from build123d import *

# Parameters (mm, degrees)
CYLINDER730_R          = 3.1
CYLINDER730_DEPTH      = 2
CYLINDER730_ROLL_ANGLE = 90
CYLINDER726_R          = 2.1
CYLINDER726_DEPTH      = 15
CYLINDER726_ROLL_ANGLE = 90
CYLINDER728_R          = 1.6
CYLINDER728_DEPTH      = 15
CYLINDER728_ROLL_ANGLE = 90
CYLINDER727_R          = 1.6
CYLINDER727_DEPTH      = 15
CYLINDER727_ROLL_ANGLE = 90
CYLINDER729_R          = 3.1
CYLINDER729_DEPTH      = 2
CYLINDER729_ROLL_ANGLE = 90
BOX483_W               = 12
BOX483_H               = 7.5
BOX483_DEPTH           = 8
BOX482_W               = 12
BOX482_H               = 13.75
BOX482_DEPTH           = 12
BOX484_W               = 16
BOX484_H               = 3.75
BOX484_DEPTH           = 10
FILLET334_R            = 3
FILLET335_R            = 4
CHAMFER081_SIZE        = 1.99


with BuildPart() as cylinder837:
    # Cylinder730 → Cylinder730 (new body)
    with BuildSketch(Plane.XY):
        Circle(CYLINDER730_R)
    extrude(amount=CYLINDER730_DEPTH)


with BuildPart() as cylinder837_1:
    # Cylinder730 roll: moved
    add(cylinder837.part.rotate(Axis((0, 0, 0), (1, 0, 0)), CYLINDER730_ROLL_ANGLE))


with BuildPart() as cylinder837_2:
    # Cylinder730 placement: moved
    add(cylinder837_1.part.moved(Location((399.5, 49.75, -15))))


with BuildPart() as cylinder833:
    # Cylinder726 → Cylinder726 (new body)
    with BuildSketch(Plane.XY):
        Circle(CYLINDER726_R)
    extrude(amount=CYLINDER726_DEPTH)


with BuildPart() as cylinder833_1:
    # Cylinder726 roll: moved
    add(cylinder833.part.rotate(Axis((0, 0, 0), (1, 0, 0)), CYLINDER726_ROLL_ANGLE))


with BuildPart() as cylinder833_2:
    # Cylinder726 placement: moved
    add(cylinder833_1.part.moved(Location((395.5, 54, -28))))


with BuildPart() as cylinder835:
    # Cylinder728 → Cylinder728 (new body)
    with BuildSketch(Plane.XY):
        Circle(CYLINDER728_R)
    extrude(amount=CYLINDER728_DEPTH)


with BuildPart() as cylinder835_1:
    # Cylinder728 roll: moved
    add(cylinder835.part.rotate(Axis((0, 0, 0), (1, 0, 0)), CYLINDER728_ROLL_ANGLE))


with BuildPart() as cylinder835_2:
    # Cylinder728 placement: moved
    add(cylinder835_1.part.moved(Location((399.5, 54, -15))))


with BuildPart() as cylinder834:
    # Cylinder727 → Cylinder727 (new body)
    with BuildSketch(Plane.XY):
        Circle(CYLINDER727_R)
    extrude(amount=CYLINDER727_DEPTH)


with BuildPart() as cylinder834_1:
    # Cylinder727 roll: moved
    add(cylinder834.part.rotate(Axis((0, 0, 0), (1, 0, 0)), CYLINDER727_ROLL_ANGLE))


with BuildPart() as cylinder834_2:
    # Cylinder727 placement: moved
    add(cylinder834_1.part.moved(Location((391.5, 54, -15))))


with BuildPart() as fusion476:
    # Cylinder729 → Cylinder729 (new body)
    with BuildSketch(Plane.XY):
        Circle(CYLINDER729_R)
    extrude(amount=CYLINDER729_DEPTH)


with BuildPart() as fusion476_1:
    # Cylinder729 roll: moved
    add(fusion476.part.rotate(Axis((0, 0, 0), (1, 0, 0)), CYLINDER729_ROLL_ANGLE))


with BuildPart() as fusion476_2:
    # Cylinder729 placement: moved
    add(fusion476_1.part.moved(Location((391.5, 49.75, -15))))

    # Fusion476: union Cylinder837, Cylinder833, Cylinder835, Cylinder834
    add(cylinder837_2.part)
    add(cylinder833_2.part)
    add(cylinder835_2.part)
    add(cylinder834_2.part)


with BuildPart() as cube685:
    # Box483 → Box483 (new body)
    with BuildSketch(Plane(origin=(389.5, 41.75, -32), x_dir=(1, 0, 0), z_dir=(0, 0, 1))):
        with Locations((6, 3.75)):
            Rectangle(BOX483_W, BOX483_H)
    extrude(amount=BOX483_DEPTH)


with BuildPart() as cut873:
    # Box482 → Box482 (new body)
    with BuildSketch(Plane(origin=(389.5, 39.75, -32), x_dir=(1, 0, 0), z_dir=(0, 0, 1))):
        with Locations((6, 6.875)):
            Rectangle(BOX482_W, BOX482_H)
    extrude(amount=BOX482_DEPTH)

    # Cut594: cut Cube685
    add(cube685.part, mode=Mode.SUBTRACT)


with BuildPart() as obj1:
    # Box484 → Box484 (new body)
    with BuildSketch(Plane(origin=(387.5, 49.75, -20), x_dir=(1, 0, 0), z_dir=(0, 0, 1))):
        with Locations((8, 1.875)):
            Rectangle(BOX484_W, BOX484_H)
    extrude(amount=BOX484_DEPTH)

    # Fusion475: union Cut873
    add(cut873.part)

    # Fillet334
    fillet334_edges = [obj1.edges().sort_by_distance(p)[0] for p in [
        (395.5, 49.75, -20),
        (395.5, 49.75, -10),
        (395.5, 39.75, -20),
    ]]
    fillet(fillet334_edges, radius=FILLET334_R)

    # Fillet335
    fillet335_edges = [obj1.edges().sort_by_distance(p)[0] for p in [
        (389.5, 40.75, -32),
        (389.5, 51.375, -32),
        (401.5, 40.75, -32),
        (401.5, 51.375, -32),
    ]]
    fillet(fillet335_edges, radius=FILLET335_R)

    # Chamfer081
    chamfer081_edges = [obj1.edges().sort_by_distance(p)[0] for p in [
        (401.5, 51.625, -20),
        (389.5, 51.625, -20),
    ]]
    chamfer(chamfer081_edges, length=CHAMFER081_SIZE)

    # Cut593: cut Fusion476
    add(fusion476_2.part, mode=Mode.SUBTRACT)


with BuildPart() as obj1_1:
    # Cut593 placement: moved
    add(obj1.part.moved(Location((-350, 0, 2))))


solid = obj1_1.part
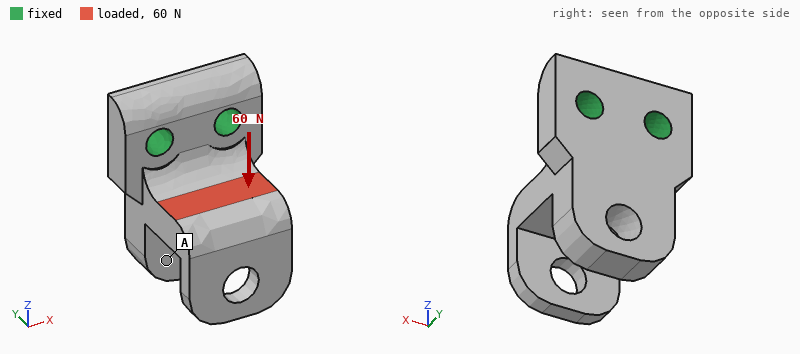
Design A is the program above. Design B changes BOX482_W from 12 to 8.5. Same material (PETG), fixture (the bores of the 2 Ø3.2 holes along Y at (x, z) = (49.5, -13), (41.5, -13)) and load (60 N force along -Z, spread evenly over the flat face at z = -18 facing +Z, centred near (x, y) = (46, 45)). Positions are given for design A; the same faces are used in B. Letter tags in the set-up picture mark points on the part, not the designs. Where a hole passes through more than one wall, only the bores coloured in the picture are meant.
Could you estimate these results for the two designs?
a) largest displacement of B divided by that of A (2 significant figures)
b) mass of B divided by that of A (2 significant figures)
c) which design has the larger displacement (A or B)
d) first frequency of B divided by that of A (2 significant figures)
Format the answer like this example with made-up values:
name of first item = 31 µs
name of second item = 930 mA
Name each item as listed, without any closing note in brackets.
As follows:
largest displacement of B divided by that of A = 1.3
mass of B divided by that of A = 0.78
which design has the larger displacement = B
first frequency of B divided by that of A = 1.1
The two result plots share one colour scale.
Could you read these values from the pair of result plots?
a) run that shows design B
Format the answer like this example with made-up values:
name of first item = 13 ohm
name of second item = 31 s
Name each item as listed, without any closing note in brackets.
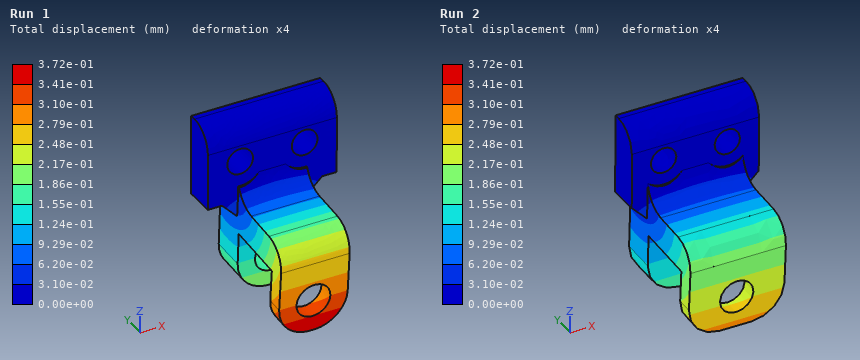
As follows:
run that shows design B = Run 1
